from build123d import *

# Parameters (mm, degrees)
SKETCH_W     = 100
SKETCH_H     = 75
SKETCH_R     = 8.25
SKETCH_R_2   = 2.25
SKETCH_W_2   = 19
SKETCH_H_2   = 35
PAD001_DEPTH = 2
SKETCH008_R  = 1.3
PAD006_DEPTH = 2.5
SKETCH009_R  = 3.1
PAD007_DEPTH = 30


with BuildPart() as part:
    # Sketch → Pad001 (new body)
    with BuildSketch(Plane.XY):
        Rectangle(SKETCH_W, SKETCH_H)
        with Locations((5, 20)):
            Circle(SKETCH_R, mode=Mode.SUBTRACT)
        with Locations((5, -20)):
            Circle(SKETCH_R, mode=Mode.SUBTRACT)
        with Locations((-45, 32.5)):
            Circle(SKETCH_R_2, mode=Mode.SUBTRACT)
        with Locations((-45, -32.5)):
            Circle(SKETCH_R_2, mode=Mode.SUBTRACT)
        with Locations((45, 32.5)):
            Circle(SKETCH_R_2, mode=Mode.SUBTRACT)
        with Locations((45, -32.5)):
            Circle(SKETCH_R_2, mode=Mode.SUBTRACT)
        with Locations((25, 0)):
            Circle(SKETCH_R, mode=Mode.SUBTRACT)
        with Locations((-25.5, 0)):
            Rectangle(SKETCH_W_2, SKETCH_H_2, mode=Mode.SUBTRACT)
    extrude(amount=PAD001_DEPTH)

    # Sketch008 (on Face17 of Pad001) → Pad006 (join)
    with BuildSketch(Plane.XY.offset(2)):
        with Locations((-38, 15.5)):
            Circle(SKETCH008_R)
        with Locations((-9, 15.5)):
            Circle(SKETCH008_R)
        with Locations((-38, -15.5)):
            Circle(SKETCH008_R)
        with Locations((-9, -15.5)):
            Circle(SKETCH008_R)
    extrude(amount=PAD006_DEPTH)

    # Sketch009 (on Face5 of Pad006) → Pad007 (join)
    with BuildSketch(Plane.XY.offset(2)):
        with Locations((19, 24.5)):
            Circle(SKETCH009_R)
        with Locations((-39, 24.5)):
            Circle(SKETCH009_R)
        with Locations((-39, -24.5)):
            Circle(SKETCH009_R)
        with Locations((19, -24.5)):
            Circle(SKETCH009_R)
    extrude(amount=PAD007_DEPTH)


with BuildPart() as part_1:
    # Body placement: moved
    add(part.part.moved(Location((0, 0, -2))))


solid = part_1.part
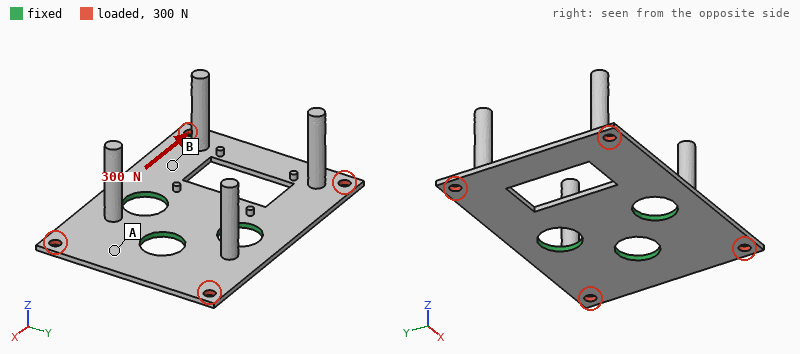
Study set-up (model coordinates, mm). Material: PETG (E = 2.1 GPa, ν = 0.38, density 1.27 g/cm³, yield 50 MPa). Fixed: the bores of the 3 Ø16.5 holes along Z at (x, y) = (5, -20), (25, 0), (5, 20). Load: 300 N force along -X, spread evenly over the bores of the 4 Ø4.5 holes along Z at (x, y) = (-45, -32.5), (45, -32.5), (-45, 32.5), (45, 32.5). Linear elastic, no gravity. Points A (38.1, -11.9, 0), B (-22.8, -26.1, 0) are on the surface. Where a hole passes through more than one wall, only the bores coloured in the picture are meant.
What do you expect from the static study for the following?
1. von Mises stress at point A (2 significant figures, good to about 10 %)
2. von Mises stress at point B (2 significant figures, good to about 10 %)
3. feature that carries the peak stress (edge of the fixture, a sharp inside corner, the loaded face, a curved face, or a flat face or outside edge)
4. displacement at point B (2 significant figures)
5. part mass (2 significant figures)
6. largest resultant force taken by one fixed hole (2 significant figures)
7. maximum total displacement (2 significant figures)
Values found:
0.52 MPa
2.0 MPa
the loaded face
20 µm
20 g
140 N
67 µm
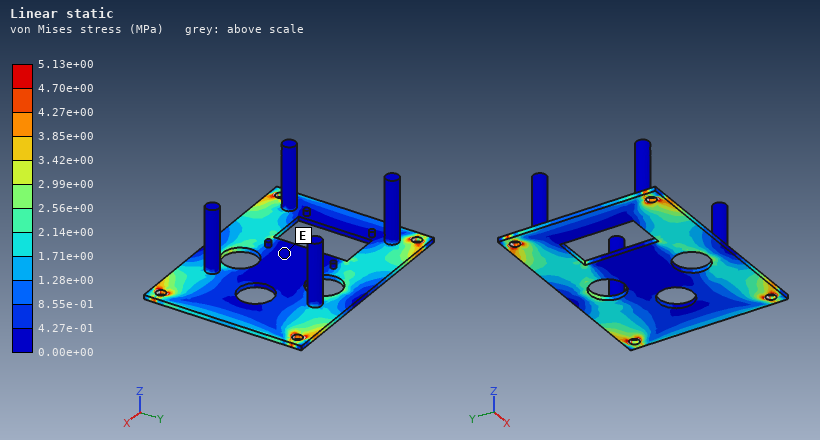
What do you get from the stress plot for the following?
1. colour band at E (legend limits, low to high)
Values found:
0.00e+00 to 4.27e-01 MPa
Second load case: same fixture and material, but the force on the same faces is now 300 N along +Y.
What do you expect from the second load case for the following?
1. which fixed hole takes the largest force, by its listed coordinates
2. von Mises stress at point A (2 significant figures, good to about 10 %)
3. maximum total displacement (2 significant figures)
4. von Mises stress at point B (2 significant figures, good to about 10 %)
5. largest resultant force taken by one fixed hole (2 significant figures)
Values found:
(25, 0)
2.2 MPa
0.41 mm
5.0 MPa
140 N
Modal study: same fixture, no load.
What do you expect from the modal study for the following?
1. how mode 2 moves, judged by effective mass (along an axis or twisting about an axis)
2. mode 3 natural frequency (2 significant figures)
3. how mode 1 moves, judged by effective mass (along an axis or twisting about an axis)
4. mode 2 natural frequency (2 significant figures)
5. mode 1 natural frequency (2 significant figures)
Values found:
twisting about X
320 Hz
along Z
190 Hz
120 Hz
